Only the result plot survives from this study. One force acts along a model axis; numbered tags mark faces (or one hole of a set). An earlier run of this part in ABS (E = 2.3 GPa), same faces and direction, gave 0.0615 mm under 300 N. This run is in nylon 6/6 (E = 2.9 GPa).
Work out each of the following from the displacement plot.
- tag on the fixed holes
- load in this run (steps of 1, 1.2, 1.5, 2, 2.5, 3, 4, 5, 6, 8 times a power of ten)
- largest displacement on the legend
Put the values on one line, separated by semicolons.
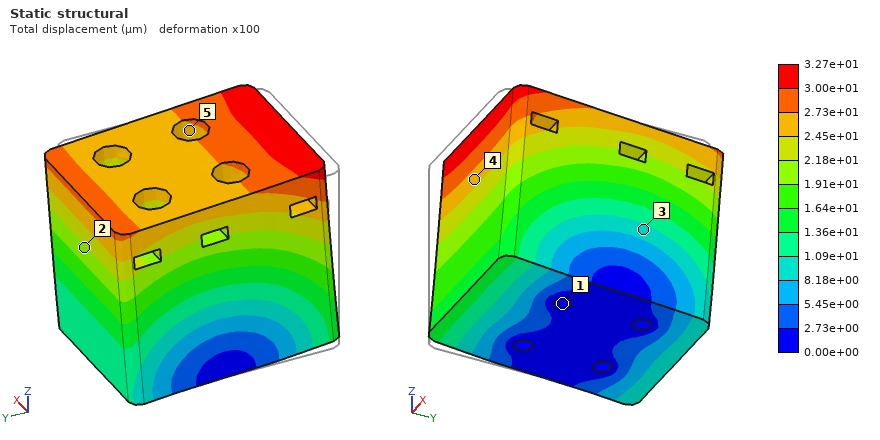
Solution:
1; 200 N; 3.27e+01 µm
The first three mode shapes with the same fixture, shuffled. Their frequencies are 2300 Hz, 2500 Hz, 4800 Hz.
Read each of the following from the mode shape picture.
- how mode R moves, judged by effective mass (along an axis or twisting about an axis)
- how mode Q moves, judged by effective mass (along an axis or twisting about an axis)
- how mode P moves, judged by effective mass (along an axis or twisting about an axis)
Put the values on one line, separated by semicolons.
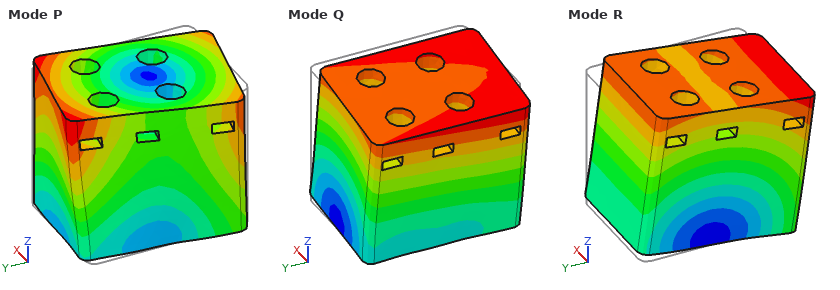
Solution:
along Y; along X; twisting about Z
